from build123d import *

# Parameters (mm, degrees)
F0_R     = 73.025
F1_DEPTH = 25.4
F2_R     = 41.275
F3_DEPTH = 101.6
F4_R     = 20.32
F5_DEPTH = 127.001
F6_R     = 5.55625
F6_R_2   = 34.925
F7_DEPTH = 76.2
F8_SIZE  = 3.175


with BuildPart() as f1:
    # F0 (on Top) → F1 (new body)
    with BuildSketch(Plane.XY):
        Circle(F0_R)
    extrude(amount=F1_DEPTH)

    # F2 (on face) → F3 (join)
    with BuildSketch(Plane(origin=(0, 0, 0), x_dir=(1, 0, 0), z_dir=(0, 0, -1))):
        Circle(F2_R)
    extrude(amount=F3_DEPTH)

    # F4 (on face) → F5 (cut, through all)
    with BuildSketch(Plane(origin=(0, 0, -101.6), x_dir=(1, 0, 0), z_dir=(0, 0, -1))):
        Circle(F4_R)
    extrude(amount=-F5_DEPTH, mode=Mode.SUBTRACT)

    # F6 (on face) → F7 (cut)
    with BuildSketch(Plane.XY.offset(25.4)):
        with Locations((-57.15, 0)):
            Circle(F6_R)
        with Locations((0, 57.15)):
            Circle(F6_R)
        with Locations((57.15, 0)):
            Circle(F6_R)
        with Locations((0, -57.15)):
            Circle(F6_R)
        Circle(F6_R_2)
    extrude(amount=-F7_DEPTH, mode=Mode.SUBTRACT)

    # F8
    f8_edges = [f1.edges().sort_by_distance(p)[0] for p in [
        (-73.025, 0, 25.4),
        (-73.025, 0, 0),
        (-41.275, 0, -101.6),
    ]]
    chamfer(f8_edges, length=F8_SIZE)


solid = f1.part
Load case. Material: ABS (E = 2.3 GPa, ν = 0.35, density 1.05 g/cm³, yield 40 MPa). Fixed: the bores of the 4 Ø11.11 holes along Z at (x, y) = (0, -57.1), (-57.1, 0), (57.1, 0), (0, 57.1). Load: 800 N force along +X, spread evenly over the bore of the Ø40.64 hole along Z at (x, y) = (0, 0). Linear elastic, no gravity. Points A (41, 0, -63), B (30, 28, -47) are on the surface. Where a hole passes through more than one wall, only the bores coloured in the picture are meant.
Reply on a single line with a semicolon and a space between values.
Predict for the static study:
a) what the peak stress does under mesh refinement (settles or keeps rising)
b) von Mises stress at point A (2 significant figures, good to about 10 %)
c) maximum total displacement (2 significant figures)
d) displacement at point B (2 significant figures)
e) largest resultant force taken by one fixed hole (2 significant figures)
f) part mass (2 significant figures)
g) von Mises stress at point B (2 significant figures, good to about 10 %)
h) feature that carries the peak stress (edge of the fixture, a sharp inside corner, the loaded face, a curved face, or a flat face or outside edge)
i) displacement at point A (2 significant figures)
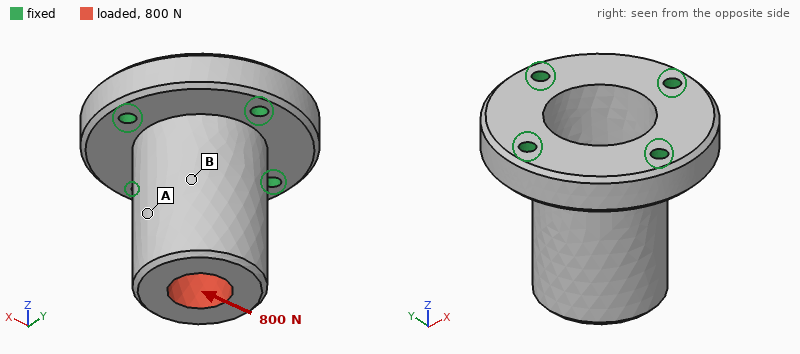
keeps rising; 0.43 MPa; 0.22 mm; 0.12 mm; 700 N; 630 g; 1.2 MPa; edge of the fixture; 0.16 mm
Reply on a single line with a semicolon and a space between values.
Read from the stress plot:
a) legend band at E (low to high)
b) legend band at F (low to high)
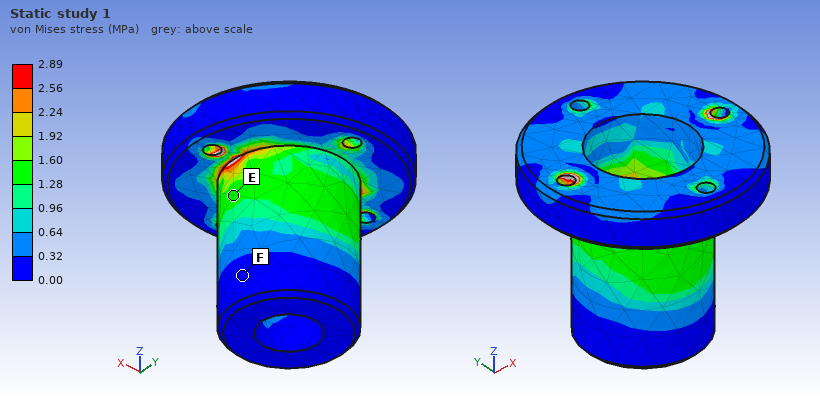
1.28 to 1.60 MPa; 0.00 to 0.32 MPa
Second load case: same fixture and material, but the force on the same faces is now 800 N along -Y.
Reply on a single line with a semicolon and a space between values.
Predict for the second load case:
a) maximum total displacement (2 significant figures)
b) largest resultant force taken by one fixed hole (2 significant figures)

0.22 mm; 700 N
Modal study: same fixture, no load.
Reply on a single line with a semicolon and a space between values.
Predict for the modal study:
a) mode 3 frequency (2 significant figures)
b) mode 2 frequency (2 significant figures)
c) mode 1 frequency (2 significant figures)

1600 Hz; 700 Hz; 700 Hz
